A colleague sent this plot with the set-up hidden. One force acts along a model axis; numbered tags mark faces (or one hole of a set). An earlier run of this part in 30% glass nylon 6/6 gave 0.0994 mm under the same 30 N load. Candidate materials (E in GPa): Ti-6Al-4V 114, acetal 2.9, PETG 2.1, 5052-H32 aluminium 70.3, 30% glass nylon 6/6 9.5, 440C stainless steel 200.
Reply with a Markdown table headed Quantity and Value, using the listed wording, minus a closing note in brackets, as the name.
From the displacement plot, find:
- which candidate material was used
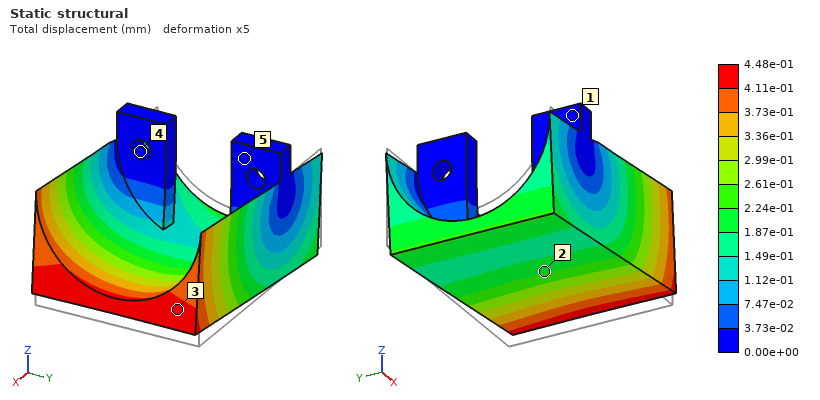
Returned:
| Quantity | Value |
|---|---|
| which candidate material was used | PETG |
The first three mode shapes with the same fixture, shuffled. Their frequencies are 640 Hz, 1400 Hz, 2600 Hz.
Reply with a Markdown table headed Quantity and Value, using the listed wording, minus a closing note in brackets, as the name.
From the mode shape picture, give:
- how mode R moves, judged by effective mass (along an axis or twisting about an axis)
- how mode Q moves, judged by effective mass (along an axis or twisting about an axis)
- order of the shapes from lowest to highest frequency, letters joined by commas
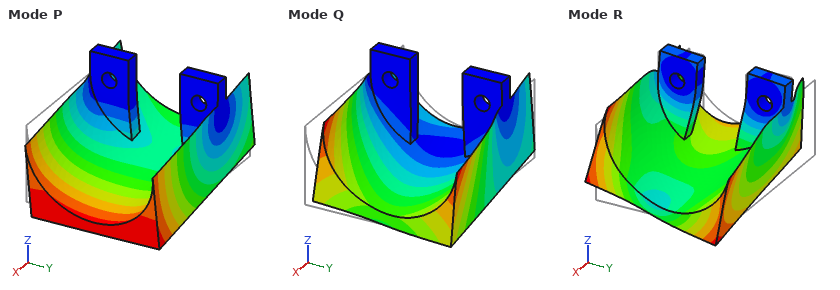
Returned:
| Quantity | Value |
|---|---|
| how mode R moves, judged by effective mass | along Y |
| how mode Q moves, judged by effective mass | along Y |
| order of the shapes from lowest to highest frequency, letters joined by commas | P, Q, R |
